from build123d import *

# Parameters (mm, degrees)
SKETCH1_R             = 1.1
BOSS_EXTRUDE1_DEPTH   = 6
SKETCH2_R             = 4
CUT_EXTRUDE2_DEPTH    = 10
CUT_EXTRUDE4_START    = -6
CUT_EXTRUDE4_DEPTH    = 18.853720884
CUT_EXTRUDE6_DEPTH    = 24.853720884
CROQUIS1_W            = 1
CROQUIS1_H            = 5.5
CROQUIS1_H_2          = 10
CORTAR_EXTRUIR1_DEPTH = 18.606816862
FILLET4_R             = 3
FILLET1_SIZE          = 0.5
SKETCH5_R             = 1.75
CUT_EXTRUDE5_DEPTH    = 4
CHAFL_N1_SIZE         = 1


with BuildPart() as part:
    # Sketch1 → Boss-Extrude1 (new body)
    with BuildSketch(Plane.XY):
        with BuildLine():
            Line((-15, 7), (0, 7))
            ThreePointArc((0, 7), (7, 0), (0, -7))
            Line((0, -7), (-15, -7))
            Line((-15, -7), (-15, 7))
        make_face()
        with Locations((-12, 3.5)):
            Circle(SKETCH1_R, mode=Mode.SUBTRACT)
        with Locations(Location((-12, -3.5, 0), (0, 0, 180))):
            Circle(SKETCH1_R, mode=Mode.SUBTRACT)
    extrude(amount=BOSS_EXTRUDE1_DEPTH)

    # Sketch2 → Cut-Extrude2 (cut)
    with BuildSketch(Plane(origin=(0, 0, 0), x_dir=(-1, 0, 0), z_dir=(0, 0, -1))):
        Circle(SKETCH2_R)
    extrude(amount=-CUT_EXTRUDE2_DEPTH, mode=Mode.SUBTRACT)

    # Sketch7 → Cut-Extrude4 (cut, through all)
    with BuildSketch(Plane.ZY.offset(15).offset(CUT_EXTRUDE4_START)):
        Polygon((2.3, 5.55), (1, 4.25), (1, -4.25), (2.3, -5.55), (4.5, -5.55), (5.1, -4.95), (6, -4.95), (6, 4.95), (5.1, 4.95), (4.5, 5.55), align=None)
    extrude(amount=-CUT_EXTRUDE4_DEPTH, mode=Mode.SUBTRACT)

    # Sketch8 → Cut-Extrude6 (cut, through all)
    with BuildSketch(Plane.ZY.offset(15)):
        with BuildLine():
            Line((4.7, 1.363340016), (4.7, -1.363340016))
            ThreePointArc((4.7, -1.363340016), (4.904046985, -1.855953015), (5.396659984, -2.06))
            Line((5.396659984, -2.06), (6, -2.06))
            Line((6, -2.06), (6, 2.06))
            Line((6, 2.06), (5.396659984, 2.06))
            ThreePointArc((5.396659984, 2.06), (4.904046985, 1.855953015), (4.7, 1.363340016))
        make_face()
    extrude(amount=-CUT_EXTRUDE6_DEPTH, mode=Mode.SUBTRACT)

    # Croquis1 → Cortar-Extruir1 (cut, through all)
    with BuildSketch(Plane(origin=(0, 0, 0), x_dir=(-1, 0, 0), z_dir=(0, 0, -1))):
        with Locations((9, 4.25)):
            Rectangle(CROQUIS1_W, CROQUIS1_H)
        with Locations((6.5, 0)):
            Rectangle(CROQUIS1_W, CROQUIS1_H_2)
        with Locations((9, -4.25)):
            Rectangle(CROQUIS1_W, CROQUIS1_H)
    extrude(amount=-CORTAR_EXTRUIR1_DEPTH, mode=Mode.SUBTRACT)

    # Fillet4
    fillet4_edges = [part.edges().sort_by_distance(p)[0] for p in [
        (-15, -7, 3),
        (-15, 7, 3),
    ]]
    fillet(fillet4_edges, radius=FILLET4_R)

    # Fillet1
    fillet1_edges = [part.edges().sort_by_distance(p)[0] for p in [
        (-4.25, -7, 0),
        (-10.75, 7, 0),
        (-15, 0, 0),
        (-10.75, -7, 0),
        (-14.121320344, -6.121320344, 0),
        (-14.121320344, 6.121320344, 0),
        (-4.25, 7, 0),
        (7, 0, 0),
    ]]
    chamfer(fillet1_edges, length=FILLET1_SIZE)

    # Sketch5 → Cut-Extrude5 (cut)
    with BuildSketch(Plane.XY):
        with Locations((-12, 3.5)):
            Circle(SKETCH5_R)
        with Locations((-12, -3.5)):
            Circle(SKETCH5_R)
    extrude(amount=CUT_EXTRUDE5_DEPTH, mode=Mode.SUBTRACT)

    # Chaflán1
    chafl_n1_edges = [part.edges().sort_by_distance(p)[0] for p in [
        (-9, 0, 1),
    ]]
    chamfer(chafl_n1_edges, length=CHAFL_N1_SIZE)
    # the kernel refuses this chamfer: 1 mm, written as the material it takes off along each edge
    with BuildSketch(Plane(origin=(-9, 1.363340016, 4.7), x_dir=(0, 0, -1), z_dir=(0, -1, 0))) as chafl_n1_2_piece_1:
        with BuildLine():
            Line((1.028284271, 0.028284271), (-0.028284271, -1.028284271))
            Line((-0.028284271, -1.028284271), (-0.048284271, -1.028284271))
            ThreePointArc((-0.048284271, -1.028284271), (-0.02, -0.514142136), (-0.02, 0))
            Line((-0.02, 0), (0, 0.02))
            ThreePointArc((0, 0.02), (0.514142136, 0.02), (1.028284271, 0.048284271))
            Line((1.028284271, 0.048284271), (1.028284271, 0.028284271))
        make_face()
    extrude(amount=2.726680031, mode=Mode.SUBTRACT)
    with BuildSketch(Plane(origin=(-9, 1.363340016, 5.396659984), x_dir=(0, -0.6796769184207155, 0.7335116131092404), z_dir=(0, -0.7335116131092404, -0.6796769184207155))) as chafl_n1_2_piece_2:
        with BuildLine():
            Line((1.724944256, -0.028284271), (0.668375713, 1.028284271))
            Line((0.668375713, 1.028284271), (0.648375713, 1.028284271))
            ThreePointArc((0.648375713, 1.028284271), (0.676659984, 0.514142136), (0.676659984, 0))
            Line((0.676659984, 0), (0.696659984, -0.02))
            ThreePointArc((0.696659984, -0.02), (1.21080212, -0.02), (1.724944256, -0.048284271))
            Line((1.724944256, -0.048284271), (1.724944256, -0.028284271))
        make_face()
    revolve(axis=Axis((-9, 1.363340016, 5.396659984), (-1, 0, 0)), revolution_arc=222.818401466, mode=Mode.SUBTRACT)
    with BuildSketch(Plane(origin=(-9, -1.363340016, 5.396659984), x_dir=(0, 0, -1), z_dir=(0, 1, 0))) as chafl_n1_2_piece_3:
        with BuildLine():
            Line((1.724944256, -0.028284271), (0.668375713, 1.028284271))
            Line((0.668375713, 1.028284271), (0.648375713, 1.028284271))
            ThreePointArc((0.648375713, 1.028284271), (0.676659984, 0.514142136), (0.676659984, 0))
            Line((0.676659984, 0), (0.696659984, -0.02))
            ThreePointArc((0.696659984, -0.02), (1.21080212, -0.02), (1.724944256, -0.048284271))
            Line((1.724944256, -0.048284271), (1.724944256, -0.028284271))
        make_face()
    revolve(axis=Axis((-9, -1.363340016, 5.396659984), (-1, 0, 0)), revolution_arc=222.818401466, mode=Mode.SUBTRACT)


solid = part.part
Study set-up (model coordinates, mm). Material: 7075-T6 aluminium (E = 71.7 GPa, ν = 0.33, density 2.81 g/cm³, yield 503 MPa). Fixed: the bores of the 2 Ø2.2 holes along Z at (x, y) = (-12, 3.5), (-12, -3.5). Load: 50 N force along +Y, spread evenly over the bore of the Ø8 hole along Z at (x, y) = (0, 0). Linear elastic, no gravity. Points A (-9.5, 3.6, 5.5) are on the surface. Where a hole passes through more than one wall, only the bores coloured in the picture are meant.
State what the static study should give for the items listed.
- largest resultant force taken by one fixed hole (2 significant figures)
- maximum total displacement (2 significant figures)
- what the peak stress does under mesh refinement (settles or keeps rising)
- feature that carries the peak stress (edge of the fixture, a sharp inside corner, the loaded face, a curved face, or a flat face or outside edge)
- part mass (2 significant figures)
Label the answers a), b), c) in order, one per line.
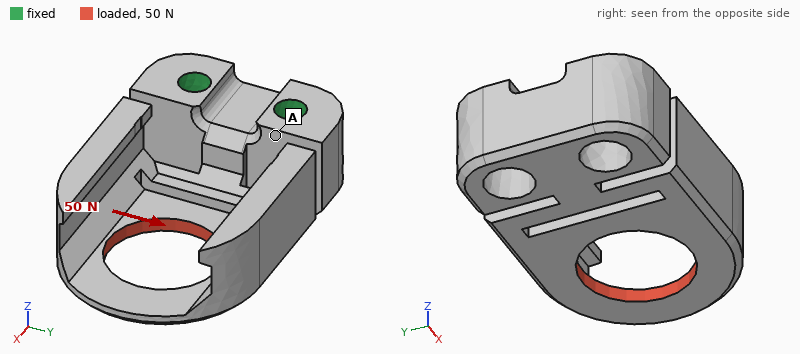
a) 73 N
b) 0.25 mm
c) keeps rising
d) a sharp inside corner
e) 1.9 g
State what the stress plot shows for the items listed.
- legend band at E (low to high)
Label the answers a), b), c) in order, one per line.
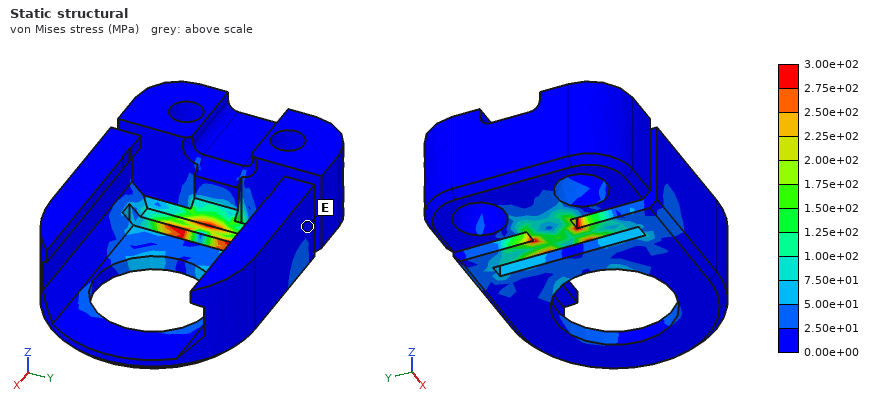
a) 0.00e+00 to 2.50e+01 MPa
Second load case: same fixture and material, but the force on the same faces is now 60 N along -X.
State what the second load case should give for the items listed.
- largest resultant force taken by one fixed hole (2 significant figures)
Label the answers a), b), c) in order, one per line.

a) 30 N
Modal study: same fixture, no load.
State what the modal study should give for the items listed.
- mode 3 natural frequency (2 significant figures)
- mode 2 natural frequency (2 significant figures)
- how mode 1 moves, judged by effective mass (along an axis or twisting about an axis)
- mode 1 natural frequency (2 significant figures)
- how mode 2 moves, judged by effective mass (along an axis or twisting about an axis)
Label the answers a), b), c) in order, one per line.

a) 3500 Hz
b) 2600 Hz
c) along Z
d) 1400 Hz
e) along Y
